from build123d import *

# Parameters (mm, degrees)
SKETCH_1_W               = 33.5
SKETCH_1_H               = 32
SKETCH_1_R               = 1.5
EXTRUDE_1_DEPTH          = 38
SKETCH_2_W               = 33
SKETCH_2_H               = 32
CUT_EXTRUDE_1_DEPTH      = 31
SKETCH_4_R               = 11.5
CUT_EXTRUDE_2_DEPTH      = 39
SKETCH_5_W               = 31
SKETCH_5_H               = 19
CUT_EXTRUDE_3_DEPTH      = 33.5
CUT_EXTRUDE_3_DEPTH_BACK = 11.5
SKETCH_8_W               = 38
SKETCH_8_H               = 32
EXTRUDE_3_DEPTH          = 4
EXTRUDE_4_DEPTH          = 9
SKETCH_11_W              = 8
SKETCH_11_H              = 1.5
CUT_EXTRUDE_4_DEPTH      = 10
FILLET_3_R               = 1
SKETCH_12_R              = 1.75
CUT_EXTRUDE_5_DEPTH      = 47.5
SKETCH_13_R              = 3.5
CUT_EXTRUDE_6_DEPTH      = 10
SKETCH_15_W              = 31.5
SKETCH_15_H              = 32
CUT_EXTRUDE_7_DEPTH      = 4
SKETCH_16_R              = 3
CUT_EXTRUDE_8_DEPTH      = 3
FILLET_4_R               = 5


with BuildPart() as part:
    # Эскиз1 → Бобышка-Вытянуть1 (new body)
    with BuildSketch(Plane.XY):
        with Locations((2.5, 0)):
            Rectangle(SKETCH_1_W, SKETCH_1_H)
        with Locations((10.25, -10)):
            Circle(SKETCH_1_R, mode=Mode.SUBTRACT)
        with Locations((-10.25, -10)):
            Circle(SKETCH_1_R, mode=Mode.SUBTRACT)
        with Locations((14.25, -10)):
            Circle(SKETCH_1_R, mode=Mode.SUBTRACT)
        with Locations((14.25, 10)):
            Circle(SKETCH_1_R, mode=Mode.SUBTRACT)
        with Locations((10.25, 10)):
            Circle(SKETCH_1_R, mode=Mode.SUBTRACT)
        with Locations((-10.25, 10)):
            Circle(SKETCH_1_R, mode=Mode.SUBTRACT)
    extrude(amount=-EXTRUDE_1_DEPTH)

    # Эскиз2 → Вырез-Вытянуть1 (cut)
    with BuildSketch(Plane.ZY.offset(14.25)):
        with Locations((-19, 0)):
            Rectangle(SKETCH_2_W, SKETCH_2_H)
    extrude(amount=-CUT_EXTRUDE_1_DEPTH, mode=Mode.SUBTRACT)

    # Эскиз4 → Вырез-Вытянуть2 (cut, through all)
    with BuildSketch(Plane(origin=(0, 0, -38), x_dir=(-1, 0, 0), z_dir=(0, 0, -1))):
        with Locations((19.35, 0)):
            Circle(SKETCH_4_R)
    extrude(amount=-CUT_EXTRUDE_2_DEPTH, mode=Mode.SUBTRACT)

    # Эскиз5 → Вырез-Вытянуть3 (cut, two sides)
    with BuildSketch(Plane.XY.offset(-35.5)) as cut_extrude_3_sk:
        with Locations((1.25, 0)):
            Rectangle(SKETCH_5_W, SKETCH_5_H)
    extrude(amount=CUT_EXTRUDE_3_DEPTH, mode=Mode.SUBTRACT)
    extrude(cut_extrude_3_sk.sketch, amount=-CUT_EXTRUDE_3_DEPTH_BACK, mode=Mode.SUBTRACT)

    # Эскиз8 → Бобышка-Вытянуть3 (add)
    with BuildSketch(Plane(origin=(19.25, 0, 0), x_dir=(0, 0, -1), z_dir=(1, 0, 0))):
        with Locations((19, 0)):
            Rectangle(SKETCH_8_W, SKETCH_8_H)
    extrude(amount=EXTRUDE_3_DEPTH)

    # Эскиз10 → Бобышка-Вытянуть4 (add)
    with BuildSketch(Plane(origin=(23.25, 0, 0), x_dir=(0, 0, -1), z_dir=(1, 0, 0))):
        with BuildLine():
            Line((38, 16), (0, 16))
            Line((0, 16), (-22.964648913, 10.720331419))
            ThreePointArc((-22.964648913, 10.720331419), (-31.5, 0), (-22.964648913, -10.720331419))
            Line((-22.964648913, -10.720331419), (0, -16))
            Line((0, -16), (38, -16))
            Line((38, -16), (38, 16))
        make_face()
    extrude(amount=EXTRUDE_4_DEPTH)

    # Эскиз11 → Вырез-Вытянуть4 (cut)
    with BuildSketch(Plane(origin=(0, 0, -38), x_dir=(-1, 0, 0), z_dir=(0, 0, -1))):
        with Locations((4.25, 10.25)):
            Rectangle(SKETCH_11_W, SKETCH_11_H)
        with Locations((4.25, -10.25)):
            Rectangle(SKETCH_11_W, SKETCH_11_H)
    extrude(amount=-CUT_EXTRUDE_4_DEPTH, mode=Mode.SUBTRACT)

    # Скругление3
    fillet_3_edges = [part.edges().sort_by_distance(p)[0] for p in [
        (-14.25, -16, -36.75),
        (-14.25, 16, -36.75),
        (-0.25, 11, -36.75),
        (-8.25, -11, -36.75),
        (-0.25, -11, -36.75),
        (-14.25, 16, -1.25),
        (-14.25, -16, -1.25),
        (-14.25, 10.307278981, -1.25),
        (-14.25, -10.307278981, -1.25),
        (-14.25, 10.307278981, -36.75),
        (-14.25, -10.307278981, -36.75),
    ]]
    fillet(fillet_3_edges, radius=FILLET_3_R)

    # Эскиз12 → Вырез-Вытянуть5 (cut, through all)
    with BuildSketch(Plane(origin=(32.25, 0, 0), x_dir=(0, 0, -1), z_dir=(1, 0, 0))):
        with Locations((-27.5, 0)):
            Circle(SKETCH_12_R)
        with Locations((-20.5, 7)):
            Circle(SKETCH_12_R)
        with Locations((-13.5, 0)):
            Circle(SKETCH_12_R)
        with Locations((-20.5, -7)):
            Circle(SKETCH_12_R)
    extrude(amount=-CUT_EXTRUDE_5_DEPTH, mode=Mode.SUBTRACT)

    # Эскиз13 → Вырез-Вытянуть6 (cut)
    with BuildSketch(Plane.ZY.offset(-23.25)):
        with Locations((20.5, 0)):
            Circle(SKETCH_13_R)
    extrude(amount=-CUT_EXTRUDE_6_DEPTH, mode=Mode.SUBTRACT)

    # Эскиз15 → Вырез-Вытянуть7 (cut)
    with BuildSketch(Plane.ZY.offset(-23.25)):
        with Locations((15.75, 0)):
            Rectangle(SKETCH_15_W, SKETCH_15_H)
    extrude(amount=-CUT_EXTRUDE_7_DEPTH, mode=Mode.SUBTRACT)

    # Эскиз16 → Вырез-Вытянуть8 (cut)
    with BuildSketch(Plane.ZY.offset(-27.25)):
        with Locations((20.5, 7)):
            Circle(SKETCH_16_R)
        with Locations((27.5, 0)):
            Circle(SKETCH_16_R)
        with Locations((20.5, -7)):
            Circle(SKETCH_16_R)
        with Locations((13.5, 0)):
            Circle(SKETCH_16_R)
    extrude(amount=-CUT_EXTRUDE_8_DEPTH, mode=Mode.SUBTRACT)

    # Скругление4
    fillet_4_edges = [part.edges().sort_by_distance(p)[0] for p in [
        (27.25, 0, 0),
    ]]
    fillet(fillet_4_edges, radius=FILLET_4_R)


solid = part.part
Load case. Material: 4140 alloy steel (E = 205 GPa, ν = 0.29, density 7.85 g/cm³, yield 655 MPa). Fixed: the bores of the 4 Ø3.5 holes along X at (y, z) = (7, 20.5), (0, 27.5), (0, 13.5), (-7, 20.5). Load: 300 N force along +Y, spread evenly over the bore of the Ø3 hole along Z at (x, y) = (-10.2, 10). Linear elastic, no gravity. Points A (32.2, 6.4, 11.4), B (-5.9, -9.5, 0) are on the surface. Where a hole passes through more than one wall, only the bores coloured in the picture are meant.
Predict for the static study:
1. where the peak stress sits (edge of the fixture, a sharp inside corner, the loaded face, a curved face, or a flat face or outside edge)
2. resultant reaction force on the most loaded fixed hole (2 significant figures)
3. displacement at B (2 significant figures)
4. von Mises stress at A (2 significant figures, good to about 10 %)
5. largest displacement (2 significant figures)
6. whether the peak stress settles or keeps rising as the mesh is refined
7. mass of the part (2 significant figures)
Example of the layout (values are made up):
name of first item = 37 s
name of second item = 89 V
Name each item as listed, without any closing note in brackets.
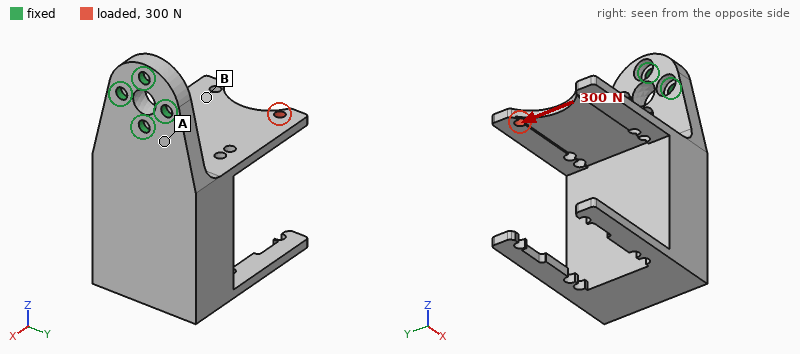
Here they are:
where the peak stress sits = edge of the fixture
resultant reaction force on the most loaded fixed hole = 720 N
displacement at B = 0.086 mm
von Mises stress at A = 58 MPa
largest displacement = 0.11 mm
whether the peak stress settles or keeps rising as the mesh is refined = keeps rising
mass of the part = 200 g
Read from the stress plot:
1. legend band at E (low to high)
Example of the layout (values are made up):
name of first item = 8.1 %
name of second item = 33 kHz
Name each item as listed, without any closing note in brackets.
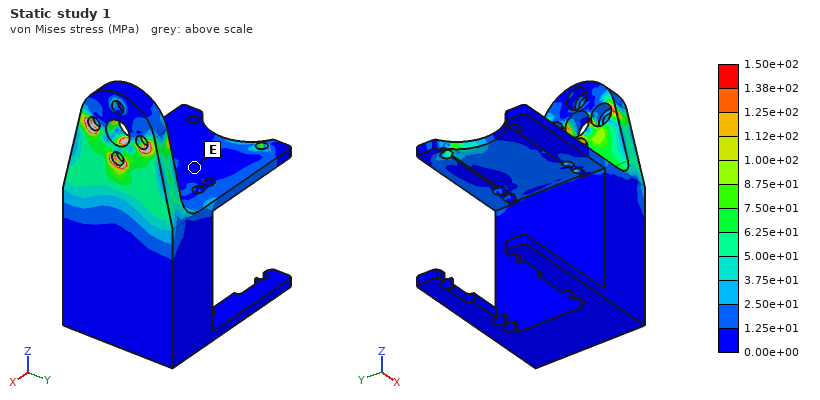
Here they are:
legend band at E = 0.00e+00 to 1.25e+01 MPa
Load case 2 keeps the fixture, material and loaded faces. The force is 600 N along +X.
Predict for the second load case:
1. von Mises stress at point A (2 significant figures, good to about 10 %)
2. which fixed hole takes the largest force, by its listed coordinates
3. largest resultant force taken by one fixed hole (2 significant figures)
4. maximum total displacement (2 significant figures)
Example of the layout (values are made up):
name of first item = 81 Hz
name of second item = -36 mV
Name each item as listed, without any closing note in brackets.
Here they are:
von Mises stress at point A = 58 MPa
which fixed hole takes the largest force, by its listed coordinates = (0, 13.5)
largest resultant force taken by one fixed hole = 1.5 kN
maximum total displacement = 0.15 mm
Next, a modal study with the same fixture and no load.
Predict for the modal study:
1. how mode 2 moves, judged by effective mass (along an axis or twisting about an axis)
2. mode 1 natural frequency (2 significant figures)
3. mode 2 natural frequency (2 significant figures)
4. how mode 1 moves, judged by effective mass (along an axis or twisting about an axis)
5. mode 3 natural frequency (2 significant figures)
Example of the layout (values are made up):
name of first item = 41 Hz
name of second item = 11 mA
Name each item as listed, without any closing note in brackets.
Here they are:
how mode 2 moves, judged by effective mass = along Y
mode 1 natural frequency = 670 Hz
mode 2 natural frequency = 1700 Hz
how mode 1 moves, judged by effective mass = along X
mode 3 natural frequency = 1900 Hz
